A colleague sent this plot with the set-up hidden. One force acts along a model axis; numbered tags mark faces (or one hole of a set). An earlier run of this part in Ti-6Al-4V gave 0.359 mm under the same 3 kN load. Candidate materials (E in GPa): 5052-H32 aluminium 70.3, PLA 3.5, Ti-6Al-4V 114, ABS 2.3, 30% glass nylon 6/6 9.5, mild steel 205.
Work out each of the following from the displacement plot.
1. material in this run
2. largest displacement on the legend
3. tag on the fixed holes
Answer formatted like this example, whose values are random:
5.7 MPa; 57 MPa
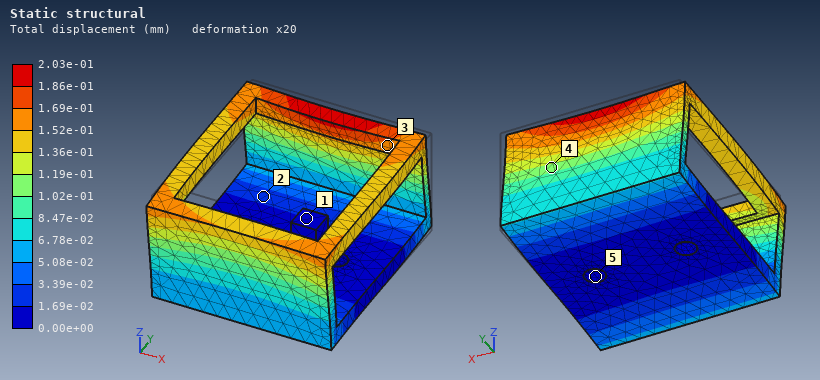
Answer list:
mild steel; 2.03e-01 mm; 5
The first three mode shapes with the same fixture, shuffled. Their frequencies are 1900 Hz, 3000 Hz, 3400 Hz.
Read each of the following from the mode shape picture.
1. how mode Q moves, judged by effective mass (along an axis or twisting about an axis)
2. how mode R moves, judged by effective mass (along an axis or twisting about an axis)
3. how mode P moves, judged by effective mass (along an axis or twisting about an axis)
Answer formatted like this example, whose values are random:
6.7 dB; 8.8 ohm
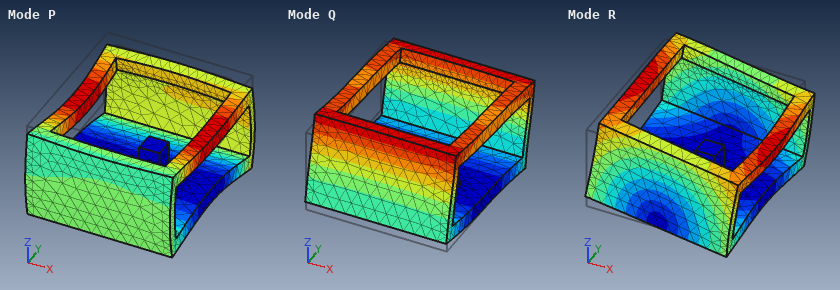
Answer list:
along Y; along X; along Z
